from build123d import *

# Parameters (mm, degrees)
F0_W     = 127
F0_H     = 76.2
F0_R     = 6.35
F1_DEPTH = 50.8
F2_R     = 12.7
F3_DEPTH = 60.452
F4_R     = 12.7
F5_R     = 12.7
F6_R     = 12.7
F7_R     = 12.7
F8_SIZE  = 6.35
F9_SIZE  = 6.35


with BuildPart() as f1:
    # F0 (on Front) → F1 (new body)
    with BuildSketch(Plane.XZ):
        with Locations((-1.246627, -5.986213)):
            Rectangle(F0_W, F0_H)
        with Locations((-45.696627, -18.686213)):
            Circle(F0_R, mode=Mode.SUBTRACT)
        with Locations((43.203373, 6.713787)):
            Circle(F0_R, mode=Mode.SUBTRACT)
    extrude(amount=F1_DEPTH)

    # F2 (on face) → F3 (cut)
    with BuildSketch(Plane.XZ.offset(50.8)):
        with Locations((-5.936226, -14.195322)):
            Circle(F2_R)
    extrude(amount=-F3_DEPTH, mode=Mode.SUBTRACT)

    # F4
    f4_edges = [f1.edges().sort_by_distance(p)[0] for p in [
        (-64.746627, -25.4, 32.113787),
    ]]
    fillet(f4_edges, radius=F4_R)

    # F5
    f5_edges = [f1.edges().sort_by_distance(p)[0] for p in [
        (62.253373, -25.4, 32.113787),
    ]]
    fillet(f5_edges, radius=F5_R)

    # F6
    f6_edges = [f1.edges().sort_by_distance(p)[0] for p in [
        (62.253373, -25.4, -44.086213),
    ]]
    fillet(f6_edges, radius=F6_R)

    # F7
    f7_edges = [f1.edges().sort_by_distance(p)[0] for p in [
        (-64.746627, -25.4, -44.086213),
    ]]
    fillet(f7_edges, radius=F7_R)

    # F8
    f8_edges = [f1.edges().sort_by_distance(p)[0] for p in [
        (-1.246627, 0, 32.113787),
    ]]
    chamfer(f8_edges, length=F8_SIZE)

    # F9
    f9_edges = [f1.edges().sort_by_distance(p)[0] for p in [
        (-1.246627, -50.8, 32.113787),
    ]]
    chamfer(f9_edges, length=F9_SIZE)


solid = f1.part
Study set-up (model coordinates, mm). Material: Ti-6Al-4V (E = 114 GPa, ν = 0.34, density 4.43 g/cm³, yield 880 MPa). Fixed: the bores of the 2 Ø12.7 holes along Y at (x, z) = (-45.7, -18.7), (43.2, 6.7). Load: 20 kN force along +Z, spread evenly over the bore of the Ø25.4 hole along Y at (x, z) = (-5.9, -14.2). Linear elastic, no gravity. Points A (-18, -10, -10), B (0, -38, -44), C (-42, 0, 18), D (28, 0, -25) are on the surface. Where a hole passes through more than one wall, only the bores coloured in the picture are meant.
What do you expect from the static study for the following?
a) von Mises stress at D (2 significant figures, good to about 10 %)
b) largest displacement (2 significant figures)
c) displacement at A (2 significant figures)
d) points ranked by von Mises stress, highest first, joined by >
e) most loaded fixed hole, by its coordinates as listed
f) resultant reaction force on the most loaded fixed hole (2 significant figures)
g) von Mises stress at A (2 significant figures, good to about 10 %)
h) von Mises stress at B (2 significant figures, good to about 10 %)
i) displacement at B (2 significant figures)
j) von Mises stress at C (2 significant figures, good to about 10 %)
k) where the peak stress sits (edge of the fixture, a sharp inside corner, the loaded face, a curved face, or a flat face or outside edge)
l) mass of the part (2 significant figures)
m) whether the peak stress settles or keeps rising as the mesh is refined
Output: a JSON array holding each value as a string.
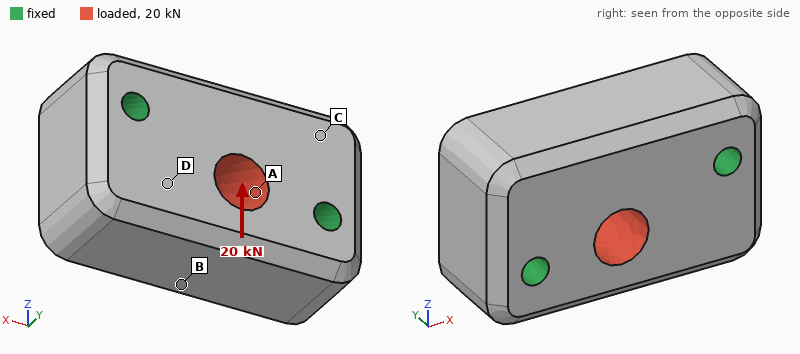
["4.0 MPa", "4.8 µm", "3.3 µm", "B > A > D > C", "(-45.7, -18.7)", "11 kN", "8.6 MPa", "11 MPa", "4.0 µm", "2.3 MPa", "edge of the fixture", "1.9 kg", "keeps rising"]
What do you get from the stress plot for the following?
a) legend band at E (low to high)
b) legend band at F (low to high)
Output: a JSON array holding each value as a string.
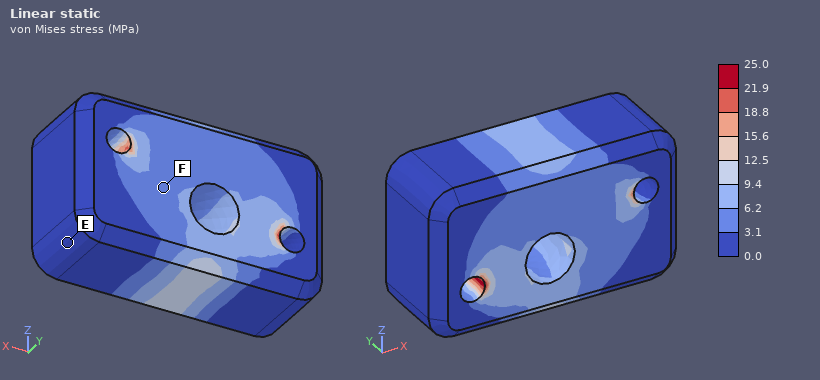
["0.0 to 3.1 MPa", "3.1 to 6.2 MPa"]
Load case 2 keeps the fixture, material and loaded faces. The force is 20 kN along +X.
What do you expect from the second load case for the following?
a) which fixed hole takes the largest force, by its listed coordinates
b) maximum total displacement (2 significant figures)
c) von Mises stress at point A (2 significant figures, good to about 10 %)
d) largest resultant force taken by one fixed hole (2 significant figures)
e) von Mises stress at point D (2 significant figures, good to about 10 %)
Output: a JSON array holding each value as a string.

["(-45.7, -18.7)", "2.8 µm", "6.6 MPa", "11 kN", "2.0 MPa"]
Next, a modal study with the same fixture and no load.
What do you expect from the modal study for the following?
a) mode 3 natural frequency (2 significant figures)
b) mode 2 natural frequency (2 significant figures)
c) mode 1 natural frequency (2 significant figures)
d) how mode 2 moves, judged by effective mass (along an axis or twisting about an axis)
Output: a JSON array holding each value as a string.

["12 kHz", "11 kHz", "9800 Hz", "along Y"]
